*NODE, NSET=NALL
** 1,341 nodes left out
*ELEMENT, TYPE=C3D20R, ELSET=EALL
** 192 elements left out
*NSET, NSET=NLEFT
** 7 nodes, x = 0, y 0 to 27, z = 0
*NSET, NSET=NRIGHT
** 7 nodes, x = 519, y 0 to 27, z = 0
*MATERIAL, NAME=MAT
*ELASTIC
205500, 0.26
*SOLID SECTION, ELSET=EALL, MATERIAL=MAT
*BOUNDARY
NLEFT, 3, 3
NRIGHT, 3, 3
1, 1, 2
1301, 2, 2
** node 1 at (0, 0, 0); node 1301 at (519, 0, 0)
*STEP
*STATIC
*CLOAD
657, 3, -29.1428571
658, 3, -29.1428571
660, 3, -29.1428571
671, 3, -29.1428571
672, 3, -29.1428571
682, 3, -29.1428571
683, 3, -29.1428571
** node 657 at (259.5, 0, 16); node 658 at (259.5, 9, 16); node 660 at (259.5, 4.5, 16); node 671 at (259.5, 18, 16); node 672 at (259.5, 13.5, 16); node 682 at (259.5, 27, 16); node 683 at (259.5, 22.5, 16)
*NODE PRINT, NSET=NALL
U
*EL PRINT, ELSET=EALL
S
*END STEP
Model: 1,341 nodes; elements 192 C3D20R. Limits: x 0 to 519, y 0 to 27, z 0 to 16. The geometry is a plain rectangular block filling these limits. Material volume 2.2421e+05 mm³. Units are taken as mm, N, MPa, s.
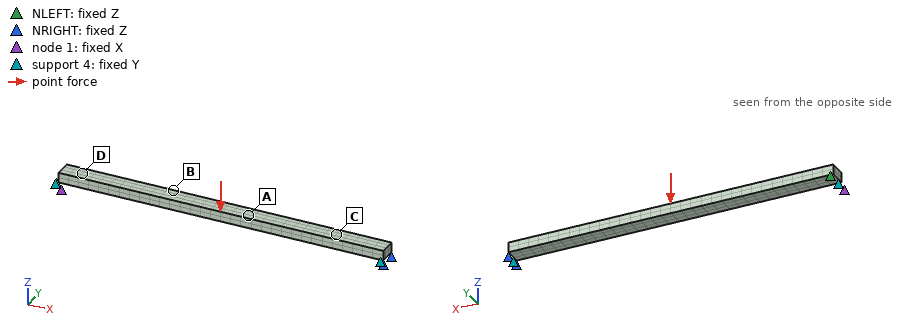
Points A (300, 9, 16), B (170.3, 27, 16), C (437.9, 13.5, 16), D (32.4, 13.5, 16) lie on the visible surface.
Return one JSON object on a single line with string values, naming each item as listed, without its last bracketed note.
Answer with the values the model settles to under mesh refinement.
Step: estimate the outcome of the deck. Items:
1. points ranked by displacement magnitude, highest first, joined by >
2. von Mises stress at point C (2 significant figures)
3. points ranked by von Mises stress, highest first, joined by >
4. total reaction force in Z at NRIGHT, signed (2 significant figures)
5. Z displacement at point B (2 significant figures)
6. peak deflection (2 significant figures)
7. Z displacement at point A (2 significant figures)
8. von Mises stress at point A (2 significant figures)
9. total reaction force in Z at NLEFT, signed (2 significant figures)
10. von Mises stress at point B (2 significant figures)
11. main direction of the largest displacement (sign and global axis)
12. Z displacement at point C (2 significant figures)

{"points ranked by displacement magnitude, highest first, joined by >": "A > B > C > D", "von Mises stress at point C": "7.2 MPa", "points ranked by von Mises stress, highest first, joined by >": "A > B > C > D", "total reaction force in Z at NRIGHT, signed": "100 N", "Z displacement at point B": "-0.27 mm", "peak deflection": "0.32 mm", "Z displacement at point A": "-0.30 mm", "von Mises stress at point A": "19 MPa", "total reaction force in Z at NLEFT, signed": "100 N", "von Mises stress at point B": "15 MPa", "main direction of the largest displacement": "-Z", "Z displacement at point C": "-0.14 mm"}
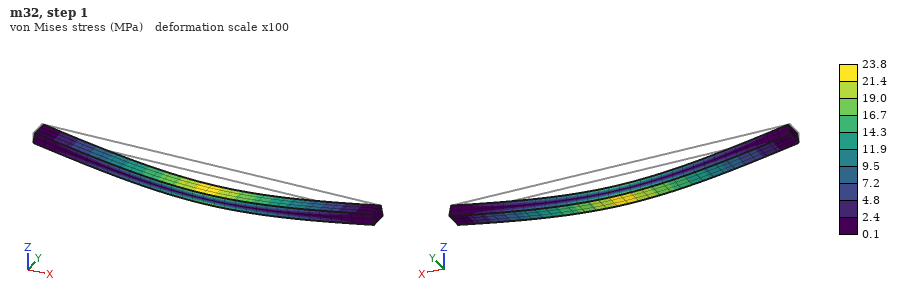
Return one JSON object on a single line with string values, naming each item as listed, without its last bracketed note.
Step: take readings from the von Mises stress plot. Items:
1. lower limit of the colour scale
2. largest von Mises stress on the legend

{"lower limit of the colour scale": "0.1 MPa", "largest von Mises stress on the legend": "23.8 MPa"}
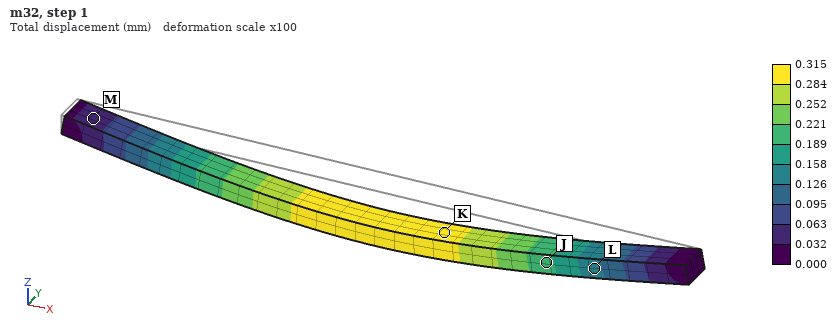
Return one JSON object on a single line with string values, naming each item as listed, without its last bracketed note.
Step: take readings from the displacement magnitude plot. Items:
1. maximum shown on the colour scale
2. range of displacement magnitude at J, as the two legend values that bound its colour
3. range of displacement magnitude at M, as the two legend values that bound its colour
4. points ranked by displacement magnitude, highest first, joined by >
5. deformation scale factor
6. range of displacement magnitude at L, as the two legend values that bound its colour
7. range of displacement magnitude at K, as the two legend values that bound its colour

{"maximum shown on the colour scale": "0.315 mm", "range of displacement magnitude at J, as the two legend values that bound its colour": "0.189 to 0.221 mm", "range of displacement magnitude at M, as the two legend values that bound its colour": "0.032 to 0.063 mm", "points ranked by displacement magnitude, highest first, joined by >": "K > J > L > M", "deformation scale factor": "100", "range of displacement magnitude at L, as the two legend values that bound its colour": "0.126 to 0.158 mm", "range of displacement magnitude at K, as the two legend values that bound its colour": "0.284 to 0.315 mm"}
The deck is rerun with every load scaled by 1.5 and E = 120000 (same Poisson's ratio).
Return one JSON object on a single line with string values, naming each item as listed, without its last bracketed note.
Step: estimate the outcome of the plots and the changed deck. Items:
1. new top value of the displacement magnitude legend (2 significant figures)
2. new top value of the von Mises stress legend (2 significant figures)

{"new top value of the displacement magnitude legend": "0.81 mm", "new top value of the von Mises stress legend": "36 MPa"}
